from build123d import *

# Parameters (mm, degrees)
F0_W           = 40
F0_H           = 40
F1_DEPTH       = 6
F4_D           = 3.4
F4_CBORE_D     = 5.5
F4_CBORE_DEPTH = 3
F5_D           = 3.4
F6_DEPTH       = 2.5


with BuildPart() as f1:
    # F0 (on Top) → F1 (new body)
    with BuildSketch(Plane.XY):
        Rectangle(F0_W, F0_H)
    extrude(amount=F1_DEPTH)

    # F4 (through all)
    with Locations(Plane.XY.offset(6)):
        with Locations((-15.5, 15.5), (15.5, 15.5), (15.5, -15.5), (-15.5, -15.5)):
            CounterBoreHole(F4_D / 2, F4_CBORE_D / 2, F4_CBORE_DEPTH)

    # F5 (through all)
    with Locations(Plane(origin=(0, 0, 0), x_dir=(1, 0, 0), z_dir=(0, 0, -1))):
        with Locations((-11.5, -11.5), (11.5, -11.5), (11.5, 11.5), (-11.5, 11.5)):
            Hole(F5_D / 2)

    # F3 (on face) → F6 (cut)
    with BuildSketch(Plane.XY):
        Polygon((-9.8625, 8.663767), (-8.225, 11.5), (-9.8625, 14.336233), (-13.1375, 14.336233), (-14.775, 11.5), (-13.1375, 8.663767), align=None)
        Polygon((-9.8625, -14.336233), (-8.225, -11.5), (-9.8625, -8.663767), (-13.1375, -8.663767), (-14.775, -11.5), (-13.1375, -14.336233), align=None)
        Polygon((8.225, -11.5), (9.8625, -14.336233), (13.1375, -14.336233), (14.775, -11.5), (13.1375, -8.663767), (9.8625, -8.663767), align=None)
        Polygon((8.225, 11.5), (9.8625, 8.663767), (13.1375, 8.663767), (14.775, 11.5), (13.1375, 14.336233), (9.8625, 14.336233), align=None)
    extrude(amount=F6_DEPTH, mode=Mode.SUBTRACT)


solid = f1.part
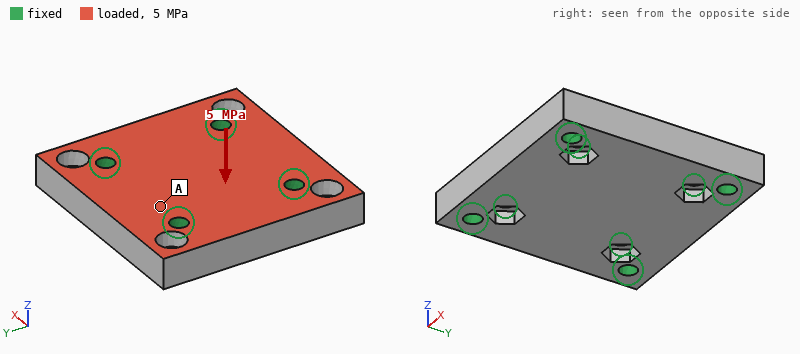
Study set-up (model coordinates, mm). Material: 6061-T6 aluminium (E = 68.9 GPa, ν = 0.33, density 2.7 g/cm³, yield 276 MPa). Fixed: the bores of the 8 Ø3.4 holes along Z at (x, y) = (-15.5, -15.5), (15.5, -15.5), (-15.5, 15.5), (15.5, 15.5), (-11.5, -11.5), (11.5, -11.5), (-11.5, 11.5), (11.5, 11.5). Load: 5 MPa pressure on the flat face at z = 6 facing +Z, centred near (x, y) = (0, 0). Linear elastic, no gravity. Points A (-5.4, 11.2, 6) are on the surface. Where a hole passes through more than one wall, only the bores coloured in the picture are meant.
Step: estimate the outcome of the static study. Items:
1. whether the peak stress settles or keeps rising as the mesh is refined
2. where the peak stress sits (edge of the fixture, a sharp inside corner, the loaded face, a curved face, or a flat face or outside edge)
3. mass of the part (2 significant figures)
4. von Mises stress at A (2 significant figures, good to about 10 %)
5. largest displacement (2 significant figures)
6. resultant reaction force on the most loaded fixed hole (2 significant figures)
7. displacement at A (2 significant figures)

keeps rising
edge of the fixture
24 g
18 MPa
12 µm
1.5 kN
7.2 µm
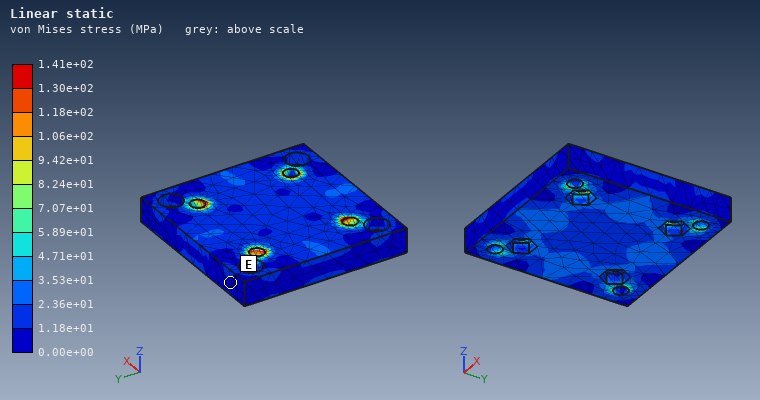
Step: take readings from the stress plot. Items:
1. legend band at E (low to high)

0.00e+00 to 1.18e+01 MPa
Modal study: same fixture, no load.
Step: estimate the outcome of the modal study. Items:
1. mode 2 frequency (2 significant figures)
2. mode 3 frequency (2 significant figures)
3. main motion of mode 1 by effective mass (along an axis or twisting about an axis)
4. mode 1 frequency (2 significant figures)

33 kHz
33 kHz
along Z
29 kHz
